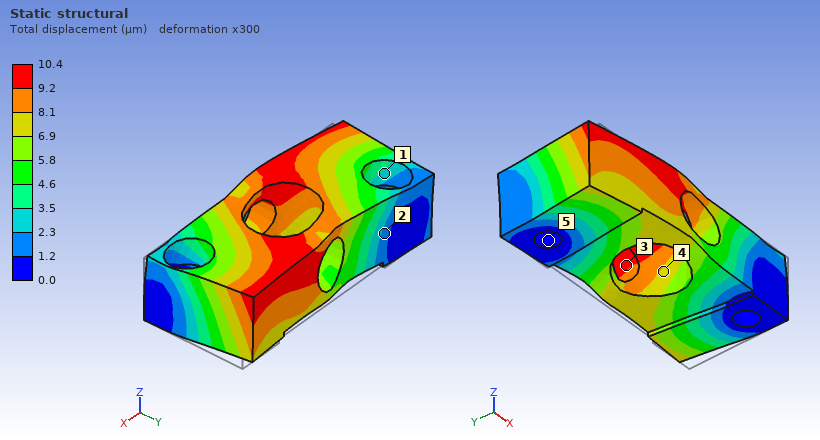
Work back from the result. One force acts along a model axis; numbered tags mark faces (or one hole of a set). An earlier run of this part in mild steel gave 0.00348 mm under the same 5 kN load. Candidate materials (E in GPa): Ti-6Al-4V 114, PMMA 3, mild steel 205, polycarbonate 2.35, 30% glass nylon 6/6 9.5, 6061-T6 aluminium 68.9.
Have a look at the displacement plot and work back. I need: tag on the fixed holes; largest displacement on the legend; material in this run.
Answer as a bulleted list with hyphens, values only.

- 5
- 10.4 µm
- 6061-T6 aluminium
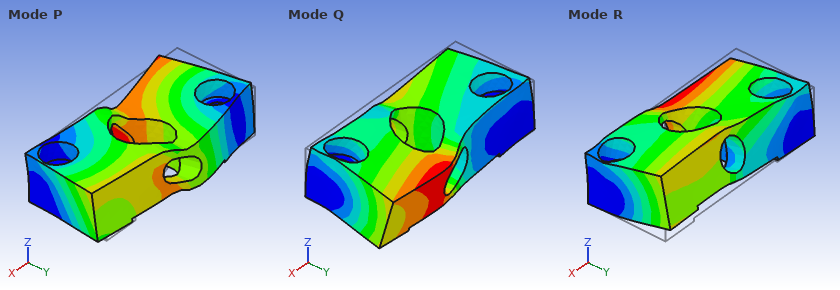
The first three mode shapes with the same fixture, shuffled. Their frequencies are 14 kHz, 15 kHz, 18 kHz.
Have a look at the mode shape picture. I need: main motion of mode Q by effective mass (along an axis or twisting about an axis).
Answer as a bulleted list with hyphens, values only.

- along Z
